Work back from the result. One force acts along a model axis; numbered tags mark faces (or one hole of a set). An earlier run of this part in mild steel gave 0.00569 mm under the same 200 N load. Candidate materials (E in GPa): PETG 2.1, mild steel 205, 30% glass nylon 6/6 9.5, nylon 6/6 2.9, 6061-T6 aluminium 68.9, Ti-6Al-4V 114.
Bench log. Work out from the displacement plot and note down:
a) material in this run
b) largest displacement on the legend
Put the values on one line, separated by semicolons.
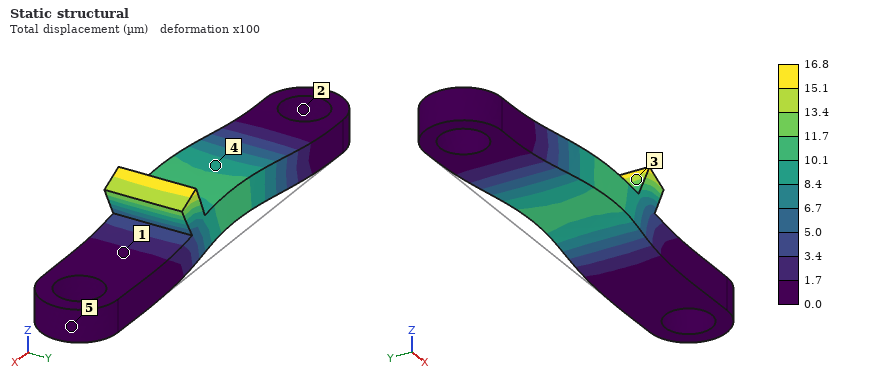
6061-T6 aluminium; 16.8 µm
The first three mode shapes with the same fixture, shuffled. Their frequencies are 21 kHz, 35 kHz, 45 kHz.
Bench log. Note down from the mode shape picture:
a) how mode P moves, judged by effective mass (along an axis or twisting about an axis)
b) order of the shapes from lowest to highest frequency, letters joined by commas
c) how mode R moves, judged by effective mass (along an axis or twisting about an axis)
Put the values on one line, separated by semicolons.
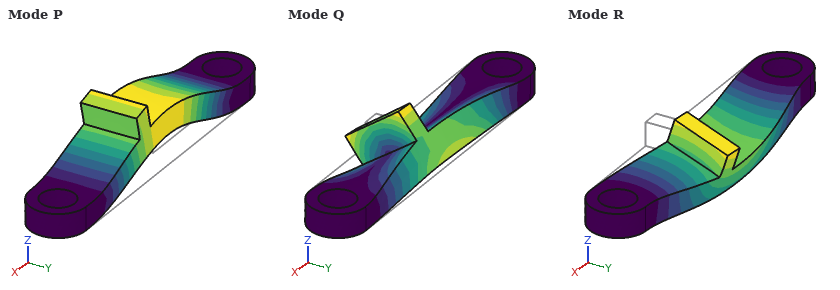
along Z; P, R, Q; along Y
